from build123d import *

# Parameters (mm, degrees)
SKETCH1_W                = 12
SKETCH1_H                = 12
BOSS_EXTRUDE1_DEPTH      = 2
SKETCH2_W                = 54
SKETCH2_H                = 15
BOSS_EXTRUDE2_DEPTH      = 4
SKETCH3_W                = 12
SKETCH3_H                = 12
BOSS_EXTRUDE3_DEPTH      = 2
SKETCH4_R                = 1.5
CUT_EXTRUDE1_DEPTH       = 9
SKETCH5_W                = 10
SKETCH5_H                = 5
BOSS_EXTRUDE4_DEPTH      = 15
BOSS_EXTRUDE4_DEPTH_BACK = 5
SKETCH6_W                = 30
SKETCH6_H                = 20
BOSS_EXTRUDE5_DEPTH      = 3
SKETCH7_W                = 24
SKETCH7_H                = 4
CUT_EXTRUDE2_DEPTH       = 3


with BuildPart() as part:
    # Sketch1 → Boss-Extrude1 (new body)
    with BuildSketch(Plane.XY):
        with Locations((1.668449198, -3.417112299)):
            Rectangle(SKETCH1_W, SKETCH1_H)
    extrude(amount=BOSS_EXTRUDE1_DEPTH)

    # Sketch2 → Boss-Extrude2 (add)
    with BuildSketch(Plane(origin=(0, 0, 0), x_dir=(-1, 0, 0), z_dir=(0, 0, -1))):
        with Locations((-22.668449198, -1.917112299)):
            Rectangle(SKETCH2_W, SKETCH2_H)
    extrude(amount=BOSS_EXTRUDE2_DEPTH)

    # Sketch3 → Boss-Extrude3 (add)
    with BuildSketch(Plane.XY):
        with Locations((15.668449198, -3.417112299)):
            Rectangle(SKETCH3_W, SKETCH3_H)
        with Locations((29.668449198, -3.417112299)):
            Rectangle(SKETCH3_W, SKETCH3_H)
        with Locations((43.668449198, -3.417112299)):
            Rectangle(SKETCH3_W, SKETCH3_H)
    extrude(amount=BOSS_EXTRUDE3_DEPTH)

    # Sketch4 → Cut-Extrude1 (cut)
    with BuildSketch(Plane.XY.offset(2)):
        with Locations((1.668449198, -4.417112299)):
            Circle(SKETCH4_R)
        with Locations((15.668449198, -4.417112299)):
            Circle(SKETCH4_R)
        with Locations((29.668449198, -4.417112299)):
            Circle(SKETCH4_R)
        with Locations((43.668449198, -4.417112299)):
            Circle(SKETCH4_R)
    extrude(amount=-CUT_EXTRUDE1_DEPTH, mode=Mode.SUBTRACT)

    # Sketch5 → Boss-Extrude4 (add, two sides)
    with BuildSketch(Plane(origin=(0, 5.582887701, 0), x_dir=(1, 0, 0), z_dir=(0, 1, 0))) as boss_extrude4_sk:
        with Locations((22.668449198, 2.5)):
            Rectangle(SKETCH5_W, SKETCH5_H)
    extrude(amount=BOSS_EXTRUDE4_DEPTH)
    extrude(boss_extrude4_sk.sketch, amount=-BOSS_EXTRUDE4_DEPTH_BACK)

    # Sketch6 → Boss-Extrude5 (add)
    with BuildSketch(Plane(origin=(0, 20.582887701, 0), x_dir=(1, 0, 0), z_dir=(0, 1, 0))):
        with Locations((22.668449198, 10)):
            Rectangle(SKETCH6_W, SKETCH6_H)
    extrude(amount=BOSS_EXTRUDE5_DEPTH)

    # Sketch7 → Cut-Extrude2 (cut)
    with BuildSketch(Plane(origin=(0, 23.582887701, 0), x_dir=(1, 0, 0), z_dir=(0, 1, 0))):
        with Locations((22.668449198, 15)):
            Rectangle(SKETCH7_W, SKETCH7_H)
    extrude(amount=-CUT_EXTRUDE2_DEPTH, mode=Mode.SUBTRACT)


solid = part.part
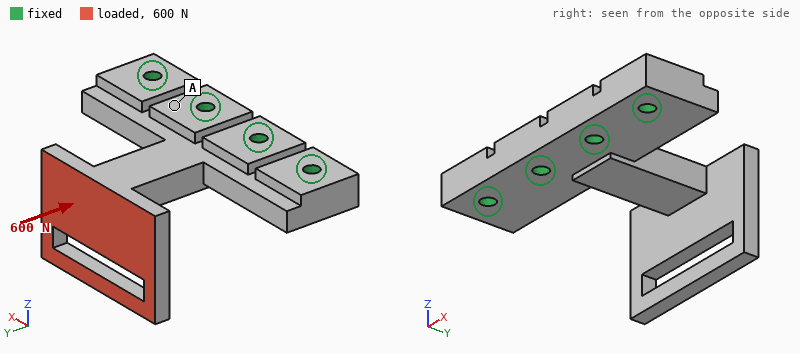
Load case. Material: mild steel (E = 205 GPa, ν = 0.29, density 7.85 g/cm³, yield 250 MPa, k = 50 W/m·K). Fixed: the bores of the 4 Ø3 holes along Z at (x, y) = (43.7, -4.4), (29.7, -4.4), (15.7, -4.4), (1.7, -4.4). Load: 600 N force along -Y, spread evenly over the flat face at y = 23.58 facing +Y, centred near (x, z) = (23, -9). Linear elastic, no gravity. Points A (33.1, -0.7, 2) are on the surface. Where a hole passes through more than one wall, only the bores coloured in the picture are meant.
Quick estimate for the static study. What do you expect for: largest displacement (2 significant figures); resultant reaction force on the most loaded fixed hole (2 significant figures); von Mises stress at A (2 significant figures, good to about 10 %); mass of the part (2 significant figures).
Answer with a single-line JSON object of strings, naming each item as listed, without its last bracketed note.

{"largest displacement": "0.13 mm", "resultant reaction force on the most loaded fixed hole": "320 N", "von Mises stress at A": "14 MPa", "mass of the part": "51 g"}
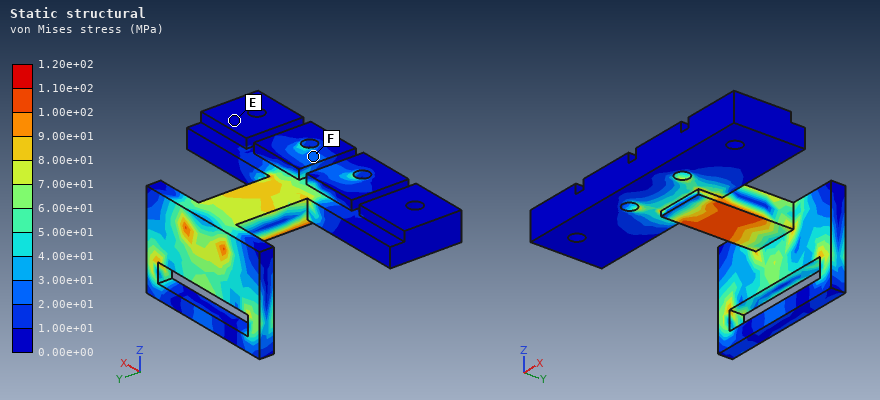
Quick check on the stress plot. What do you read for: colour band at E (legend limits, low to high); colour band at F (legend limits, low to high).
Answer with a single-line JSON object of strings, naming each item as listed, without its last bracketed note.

{"colour band at E": "0.00e+00 to 1.00e+01 MPa", "colour band at F": "2.00e+01 to 3.00e+01 MPa"}
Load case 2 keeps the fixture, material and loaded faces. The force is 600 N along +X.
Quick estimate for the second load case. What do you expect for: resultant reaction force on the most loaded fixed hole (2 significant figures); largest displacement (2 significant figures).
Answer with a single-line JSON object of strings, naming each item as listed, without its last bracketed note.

{"resultant reaction force on the most loaded fixed hole": "870 N", "largest displacement": "100 µm"}
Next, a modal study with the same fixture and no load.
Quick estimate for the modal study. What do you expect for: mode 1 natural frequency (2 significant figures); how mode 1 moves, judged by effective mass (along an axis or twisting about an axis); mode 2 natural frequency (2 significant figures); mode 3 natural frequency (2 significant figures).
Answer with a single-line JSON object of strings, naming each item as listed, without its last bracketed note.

{"mode 1 natural frequency": "2700 Hz", "how mode 1 moves, judged by effective mass": "along Z", "mode 2 natural frequency": "3900 Hz", "mode 3 natural frequency": "6100 Hz"}
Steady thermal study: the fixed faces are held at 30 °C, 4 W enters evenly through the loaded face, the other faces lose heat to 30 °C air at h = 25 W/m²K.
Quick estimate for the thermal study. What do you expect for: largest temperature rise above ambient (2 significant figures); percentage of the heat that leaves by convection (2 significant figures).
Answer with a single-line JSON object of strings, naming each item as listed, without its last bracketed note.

{"largest temperature rise above ambient": "40 K", "percentage of the heat that leaves by convection": "25 %"}
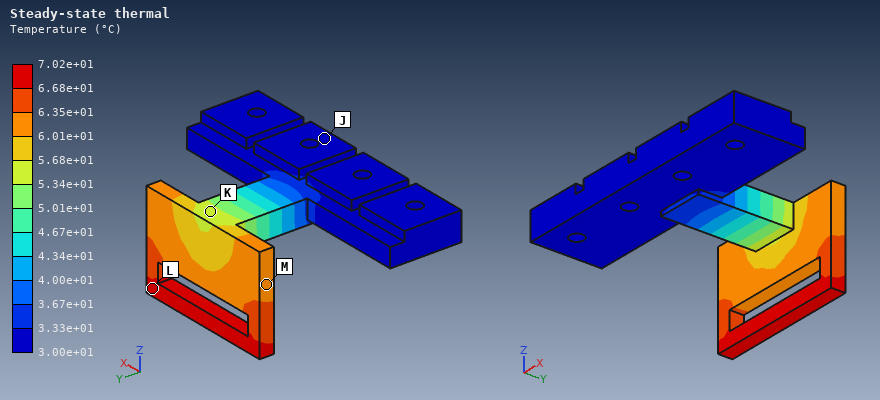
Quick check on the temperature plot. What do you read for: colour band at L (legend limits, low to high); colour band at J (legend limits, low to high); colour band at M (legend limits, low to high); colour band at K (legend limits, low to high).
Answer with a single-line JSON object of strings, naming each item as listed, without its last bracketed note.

{"colour band at L": "6.68e+01 to 7.02e+01 °C", "colour band at J": "3.00e+01 to 3.33e+01 °C", "colour band at M": "6.01e+01 to 6.35e+01 °C", "colour band at K": "5.34e+01 to 5.68e+01 °C"}
